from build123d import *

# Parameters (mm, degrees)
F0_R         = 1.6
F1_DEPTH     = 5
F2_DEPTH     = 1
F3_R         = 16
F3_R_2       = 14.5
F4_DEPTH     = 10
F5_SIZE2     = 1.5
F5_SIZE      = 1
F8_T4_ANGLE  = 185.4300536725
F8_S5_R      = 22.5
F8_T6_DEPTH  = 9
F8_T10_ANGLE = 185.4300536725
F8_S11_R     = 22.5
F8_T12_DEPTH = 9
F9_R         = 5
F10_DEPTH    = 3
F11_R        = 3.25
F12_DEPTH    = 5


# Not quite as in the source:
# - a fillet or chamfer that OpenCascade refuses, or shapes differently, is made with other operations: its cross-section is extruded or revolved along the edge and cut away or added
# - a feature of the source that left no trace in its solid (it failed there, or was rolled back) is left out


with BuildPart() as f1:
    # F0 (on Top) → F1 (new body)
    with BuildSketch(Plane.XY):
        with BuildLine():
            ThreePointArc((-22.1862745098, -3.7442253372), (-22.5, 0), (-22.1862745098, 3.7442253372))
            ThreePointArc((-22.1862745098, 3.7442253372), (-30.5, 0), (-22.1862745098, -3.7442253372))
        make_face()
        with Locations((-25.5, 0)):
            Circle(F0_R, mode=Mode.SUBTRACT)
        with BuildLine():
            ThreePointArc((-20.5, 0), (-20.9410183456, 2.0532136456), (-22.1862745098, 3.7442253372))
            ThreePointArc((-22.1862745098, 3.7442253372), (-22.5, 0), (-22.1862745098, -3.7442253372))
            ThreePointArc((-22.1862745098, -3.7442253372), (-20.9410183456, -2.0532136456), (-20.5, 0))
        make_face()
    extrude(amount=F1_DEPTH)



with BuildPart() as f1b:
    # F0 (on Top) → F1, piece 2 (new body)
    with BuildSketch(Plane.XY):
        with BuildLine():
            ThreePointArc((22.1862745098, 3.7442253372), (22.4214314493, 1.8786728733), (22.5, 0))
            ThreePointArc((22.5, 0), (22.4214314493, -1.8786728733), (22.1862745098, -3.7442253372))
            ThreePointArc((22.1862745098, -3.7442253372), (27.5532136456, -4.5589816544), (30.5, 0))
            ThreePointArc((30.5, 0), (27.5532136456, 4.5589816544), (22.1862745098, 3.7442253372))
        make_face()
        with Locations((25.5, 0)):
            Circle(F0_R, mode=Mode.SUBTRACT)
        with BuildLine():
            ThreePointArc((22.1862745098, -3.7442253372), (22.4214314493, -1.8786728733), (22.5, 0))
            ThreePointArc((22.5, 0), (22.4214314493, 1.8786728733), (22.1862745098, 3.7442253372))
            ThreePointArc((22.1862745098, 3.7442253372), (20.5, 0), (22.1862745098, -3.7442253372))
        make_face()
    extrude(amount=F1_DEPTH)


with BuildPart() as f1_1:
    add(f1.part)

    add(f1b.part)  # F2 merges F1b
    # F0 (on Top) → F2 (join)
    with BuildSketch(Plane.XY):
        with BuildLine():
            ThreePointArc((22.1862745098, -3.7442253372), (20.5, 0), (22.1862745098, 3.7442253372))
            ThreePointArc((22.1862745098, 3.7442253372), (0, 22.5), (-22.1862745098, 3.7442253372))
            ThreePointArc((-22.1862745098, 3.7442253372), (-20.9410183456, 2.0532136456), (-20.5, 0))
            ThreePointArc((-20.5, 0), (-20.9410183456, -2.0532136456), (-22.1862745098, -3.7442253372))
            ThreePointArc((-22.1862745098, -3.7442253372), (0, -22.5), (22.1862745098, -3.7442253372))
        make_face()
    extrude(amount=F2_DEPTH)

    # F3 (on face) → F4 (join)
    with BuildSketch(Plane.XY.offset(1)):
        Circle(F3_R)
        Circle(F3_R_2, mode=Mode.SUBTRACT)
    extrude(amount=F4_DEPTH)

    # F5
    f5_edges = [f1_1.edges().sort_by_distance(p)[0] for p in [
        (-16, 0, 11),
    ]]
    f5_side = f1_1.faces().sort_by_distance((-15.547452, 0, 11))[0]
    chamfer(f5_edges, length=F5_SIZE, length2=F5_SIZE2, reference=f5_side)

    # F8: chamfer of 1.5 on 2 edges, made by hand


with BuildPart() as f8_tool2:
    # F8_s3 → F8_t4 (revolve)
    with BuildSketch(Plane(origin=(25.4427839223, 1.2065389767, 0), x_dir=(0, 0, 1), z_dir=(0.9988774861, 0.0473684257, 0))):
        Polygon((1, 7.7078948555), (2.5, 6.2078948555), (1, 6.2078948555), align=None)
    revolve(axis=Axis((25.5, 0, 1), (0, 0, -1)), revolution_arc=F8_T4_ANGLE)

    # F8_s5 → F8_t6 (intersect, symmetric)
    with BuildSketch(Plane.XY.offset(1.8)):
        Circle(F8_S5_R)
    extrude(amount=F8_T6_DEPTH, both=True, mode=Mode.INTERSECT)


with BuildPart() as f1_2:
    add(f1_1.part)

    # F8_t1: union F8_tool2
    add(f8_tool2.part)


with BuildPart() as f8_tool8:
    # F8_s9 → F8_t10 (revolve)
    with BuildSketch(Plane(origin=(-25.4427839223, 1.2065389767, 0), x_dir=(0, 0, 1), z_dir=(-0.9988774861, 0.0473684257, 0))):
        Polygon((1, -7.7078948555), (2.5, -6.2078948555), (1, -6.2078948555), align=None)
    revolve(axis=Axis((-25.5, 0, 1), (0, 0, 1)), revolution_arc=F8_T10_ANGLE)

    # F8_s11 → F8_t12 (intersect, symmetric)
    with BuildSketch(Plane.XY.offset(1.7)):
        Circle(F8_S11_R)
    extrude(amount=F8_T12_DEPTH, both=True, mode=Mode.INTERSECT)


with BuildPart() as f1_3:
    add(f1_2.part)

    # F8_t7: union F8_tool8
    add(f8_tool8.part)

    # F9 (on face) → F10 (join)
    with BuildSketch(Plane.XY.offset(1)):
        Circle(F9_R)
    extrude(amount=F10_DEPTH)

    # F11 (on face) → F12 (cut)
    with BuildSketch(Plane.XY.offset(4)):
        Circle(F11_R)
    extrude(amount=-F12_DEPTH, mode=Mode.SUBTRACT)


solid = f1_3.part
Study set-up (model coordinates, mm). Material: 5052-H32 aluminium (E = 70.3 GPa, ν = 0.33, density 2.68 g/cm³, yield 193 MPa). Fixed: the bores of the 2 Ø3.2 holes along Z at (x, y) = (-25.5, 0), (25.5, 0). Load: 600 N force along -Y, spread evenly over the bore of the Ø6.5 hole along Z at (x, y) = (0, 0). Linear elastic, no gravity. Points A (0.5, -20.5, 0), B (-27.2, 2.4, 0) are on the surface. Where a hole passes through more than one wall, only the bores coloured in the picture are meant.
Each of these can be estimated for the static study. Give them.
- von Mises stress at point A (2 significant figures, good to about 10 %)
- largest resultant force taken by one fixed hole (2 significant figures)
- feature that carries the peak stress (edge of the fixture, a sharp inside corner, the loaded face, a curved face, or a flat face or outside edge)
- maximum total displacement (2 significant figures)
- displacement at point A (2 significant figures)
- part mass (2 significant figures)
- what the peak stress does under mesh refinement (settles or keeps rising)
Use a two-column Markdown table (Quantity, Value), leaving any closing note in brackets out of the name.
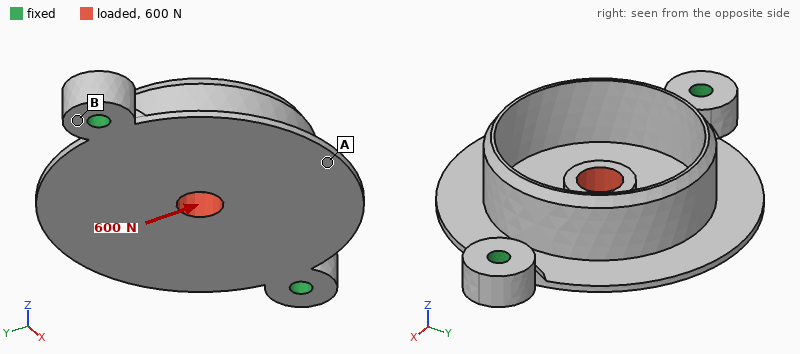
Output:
| Quantity | Value |
|---|---|
| von Mises stress at point A | 16 MPa |
| largest resultant force taken by one fixed hole | 300 N |
| feature that carries the peak stress | a sharp inside corner |
| maximum total displacement | 0.13 mm |
| displacement at point A | 0.12 mm |
| part mass | 10 g |
| what the peak stress does under mesh refinement | keeps rising |
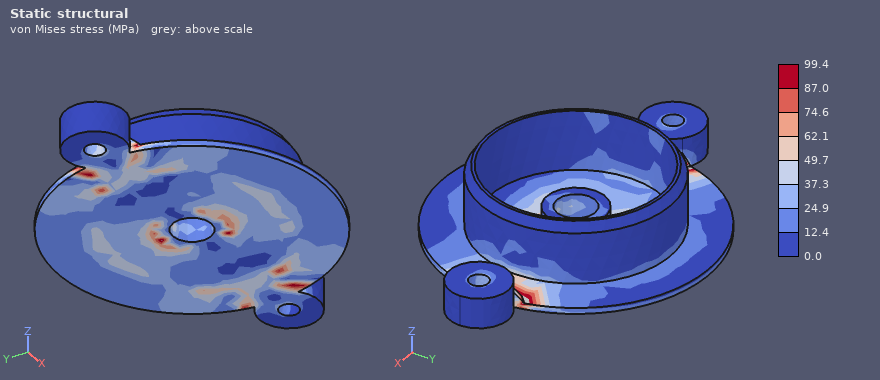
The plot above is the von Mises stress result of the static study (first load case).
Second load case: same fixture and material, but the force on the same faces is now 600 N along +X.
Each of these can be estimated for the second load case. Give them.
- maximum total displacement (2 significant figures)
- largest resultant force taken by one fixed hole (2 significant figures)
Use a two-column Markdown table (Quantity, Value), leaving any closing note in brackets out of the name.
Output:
| Quantity | Value |
|---|---|
| maximum total displacement | 35 µm |
| largest resultant force taken by one fixed hole | 300 N |
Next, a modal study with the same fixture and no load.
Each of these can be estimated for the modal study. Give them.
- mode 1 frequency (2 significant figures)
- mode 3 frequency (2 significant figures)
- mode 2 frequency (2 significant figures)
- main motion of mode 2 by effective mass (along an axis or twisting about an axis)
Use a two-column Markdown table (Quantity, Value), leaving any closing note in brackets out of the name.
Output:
| Quantity | Value |
|---|---|
| mode 1 frequency | 1800 Hz |
| mode 3 frequency | 6900 Hz |
| mode 2 frequency | 3200 Hz |
| main motion of mode 2 by effective mass | along Z |
